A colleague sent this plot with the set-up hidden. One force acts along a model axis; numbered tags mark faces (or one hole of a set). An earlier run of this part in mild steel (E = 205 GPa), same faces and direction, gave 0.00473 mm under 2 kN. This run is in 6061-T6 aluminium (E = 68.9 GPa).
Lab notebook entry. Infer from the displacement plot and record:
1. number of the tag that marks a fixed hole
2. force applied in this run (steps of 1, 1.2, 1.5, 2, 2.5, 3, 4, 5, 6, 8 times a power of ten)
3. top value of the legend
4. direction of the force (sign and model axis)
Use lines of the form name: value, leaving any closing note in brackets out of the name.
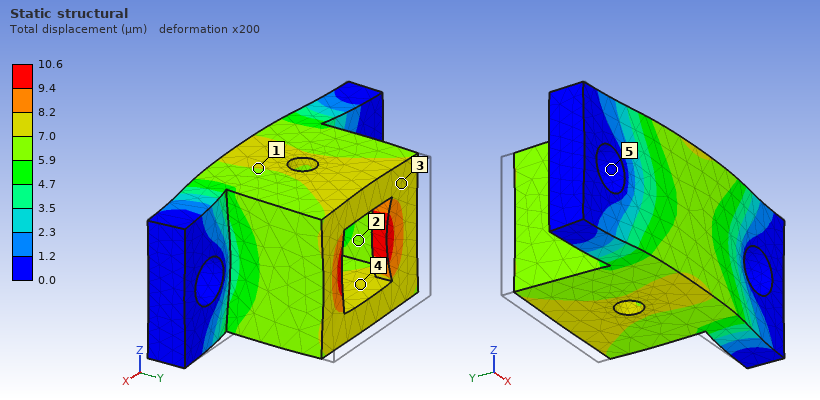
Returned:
number of the tag that marks a fixed hole: 5
force applied in this run: 1.5 kN
top value of the legend: 10.6 µm
direction of the force: -Y
